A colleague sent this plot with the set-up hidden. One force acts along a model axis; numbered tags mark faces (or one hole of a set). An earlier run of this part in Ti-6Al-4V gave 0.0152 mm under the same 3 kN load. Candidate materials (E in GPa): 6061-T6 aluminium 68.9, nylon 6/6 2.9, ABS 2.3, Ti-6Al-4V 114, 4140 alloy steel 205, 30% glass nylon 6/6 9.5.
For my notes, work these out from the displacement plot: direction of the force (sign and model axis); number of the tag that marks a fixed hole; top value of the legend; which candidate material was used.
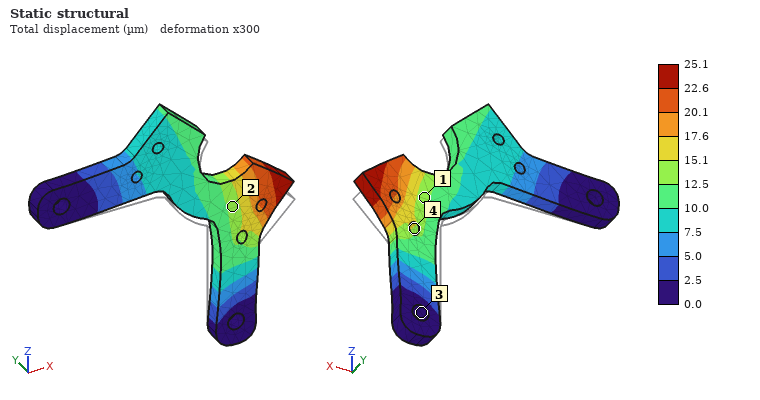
+Z
3
25.1 µm
6061-T6 aluminium
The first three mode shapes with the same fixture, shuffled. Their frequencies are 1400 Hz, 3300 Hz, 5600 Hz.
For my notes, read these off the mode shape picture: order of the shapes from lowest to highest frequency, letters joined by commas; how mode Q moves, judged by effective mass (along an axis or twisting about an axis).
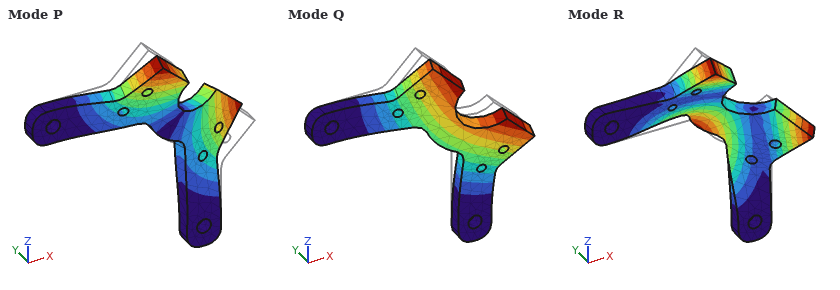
Q, P, R
along Y
